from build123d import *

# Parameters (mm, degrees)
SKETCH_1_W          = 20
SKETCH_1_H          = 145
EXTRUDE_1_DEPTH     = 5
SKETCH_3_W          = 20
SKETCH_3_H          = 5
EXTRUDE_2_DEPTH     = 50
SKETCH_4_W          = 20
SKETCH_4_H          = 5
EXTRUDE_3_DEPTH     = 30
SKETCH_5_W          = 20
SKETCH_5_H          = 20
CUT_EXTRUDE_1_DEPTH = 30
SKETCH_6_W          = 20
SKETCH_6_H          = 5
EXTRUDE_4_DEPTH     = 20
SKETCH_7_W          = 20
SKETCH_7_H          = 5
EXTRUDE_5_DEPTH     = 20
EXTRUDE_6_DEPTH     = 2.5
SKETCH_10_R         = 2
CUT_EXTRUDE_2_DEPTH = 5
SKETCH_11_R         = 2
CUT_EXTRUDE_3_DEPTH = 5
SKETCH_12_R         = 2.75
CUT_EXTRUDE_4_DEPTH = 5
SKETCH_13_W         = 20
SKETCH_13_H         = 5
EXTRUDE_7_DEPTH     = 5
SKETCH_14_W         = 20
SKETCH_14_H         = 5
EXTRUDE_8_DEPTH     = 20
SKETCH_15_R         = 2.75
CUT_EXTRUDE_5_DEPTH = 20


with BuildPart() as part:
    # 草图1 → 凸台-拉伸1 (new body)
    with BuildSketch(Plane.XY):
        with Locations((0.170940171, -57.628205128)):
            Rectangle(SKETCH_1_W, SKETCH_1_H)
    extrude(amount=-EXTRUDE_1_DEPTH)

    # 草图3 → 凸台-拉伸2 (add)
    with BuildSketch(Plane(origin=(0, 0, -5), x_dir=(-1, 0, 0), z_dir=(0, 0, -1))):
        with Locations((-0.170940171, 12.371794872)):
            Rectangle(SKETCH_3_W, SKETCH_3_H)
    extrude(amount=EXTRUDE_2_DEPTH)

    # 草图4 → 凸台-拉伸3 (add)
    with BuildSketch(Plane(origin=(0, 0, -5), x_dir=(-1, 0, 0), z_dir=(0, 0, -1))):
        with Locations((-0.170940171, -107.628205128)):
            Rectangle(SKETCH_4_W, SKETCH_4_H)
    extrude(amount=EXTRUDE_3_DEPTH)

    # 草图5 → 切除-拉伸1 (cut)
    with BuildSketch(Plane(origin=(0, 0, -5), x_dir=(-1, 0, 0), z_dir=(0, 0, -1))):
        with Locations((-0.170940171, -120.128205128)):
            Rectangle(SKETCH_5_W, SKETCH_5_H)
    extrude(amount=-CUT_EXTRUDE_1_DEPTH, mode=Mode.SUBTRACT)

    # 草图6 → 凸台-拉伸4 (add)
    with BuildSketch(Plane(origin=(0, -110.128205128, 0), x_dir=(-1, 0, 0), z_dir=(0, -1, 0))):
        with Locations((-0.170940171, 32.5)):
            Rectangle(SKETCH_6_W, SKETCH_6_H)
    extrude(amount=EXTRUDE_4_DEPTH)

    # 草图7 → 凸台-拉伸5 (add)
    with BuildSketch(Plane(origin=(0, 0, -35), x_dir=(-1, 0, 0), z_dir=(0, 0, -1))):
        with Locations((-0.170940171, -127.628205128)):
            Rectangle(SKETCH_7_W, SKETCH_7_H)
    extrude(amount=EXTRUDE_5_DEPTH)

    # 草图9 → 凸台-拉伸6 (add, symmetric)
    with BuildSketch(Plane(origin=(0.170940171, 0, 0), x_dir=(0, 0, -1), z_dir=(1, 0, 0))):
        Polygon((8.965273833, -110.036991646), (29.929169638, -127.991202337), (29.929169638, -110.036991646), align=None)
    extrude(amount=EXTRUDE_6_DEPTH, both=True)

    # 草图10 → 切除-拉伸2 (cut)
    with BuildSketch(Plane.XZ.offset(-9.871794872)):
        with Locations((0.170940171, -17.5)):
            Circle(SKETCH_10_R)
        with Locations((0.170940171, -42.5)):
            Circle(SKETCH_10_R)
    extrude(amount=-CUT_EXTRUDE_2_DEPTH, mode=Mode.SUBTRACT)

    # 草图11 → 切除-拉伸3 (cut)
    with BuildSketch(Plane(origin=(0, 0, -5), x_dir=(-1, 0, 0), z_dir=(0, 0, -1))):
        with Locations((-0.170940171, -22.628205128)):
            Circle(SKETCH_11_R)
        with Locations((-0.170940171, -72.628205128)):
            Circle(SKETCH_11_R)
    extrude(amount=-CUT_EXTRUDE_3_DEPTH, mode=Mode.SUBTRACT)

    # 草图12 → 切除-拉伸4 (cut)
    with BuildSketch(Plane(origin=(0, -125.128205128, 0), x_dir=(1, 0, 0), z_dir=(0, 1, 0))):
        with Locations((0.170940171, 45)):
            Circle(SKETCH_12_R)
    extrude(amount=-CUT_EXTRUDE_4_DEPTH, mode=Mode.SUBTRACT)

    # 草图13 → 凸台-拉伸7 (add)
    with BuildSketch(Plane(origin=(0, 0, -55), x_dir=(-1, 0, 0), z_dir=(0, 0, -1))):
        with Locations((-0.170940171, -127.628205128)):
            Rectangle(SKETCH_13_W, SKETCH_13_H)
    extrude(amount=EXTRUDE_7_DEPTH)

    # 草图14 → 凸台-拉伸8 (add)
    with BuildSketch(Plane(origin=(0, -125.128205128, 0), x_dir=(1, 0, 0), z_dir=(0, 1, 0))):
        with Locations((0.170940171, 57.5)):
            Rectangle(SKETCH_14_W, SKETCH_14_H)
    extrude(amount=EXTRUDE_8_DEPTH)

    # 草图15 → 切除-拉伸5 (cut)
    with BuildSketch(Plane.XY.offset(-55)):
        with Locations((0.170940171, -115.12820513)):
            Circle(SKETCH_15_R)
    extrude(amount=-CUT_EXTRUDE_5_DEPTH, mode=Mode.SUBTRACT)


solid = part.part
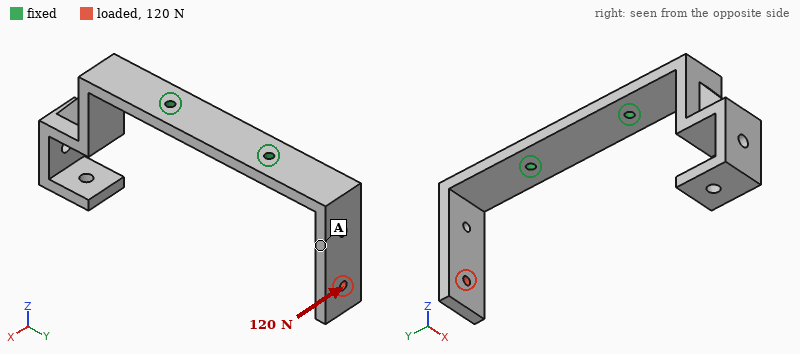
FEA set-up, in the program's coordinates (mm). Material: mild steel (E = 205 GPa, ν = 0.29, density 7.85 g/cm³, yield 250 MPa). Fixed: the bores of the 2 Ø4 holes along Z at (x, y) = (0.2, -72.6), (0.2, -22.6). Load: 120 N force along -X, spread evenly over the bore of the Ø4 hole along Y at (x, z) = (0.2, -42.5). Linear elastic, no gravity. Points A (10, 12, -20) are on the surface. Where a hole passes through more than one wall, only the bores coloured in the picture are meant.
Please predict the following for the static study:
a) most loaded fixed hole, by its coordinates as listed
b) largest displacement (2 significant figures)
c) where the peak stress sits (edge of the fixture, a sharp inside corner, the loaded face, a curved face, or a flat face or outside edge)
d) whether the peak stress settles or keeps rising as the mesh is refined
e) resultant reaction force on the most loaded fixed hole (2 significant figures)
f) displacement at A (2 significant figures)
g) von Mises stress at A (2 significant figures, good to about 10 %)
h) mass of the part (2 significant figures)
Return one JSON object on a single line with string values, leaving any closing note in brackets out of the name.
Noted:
{"most loaded fixed hole, by its coordinates as listed": "(0.2, -22.6)", "largest displacement": "0.16 mm", "where the peak stress sits": "edge of the fixture", "whether the peak stress settles or keeps rising as the mesh is refined": "keeps rising", "resultant reaction force on the most loaded fixed hole": "180 N", "displacement at A": "0.059 mm", "von Mises stress at A": "7.8 MPa", "mass of the part": "220 g"}
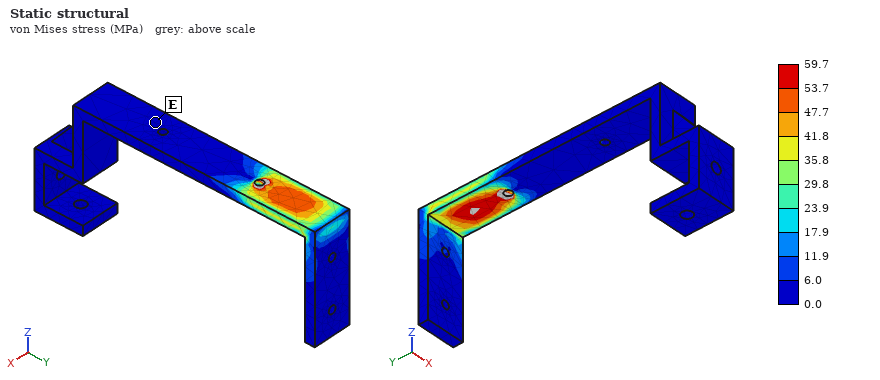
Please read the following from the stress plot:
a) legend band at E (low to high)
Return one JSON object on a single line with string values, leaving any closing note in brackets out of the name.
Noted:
{"legend band at E": "0.0 to 6.0 MPa"}
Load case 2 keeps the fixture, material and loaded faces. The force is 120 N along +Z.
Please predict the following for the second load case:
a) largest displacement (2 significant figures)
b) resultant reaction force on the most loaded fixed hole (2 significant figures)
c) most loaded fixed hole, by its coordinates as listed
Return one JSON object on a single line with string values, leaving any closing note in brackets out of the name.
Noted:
{"largest displacement": "0.10 mm", "resultant reaction force on the most loaded fixed hole": "130 N", "most loaded fixed hole, by its coordinates as listed": "(0.2, -22.6)"}
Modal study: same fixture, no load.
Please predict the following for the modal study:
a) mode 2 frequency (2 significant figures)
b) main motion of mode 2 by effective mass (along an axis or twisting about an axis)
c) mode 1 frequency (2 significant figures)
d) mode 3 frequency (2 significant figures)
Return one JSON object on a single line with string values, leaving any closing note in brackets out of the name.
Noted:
{"mode 2 frequency": "590 Hz", "main motion of mode 2 by effective mass": "along X", "mode 1 frequency": "380 Hz", "mode 3 frequency": "710 Hz"}
